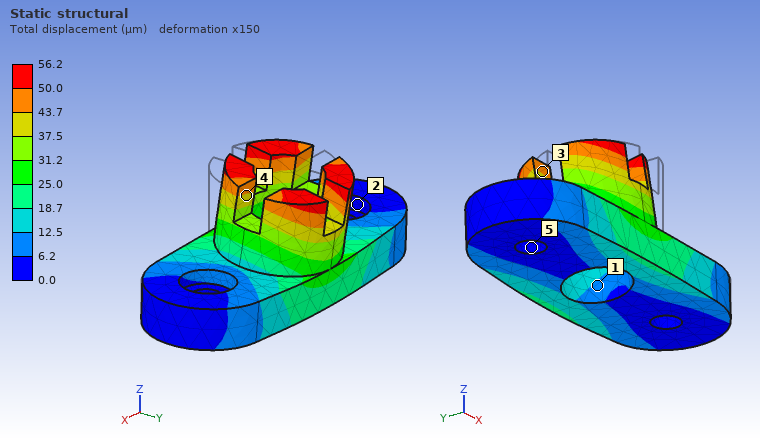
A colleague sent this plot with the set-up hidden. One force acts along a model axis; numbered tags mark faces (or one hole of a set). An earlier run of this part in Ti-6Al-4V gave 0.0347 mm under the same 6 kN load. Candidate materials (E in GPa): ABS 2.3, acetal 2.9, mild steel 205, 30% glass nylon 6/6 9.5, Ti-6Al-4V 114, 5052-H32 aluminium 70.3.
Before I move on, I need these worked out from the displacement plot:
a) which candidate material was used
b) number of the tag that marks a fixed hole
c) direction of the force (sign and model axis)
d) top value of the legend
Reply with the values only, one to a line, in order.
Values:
5052-H32 aluminium
5
+Y
56.2 µm
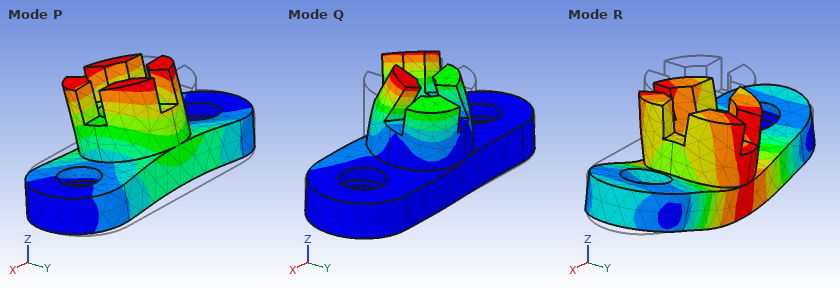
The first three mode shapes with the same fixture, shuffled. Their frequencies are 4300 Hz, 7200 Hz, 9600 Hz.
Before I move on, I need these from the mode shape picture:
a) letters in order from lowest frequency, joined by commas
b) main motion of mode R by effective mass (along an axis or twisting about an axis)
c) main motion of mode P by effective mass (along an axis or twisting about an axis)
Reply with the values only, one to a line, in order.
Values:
P, R, Q
along Z
along Y
